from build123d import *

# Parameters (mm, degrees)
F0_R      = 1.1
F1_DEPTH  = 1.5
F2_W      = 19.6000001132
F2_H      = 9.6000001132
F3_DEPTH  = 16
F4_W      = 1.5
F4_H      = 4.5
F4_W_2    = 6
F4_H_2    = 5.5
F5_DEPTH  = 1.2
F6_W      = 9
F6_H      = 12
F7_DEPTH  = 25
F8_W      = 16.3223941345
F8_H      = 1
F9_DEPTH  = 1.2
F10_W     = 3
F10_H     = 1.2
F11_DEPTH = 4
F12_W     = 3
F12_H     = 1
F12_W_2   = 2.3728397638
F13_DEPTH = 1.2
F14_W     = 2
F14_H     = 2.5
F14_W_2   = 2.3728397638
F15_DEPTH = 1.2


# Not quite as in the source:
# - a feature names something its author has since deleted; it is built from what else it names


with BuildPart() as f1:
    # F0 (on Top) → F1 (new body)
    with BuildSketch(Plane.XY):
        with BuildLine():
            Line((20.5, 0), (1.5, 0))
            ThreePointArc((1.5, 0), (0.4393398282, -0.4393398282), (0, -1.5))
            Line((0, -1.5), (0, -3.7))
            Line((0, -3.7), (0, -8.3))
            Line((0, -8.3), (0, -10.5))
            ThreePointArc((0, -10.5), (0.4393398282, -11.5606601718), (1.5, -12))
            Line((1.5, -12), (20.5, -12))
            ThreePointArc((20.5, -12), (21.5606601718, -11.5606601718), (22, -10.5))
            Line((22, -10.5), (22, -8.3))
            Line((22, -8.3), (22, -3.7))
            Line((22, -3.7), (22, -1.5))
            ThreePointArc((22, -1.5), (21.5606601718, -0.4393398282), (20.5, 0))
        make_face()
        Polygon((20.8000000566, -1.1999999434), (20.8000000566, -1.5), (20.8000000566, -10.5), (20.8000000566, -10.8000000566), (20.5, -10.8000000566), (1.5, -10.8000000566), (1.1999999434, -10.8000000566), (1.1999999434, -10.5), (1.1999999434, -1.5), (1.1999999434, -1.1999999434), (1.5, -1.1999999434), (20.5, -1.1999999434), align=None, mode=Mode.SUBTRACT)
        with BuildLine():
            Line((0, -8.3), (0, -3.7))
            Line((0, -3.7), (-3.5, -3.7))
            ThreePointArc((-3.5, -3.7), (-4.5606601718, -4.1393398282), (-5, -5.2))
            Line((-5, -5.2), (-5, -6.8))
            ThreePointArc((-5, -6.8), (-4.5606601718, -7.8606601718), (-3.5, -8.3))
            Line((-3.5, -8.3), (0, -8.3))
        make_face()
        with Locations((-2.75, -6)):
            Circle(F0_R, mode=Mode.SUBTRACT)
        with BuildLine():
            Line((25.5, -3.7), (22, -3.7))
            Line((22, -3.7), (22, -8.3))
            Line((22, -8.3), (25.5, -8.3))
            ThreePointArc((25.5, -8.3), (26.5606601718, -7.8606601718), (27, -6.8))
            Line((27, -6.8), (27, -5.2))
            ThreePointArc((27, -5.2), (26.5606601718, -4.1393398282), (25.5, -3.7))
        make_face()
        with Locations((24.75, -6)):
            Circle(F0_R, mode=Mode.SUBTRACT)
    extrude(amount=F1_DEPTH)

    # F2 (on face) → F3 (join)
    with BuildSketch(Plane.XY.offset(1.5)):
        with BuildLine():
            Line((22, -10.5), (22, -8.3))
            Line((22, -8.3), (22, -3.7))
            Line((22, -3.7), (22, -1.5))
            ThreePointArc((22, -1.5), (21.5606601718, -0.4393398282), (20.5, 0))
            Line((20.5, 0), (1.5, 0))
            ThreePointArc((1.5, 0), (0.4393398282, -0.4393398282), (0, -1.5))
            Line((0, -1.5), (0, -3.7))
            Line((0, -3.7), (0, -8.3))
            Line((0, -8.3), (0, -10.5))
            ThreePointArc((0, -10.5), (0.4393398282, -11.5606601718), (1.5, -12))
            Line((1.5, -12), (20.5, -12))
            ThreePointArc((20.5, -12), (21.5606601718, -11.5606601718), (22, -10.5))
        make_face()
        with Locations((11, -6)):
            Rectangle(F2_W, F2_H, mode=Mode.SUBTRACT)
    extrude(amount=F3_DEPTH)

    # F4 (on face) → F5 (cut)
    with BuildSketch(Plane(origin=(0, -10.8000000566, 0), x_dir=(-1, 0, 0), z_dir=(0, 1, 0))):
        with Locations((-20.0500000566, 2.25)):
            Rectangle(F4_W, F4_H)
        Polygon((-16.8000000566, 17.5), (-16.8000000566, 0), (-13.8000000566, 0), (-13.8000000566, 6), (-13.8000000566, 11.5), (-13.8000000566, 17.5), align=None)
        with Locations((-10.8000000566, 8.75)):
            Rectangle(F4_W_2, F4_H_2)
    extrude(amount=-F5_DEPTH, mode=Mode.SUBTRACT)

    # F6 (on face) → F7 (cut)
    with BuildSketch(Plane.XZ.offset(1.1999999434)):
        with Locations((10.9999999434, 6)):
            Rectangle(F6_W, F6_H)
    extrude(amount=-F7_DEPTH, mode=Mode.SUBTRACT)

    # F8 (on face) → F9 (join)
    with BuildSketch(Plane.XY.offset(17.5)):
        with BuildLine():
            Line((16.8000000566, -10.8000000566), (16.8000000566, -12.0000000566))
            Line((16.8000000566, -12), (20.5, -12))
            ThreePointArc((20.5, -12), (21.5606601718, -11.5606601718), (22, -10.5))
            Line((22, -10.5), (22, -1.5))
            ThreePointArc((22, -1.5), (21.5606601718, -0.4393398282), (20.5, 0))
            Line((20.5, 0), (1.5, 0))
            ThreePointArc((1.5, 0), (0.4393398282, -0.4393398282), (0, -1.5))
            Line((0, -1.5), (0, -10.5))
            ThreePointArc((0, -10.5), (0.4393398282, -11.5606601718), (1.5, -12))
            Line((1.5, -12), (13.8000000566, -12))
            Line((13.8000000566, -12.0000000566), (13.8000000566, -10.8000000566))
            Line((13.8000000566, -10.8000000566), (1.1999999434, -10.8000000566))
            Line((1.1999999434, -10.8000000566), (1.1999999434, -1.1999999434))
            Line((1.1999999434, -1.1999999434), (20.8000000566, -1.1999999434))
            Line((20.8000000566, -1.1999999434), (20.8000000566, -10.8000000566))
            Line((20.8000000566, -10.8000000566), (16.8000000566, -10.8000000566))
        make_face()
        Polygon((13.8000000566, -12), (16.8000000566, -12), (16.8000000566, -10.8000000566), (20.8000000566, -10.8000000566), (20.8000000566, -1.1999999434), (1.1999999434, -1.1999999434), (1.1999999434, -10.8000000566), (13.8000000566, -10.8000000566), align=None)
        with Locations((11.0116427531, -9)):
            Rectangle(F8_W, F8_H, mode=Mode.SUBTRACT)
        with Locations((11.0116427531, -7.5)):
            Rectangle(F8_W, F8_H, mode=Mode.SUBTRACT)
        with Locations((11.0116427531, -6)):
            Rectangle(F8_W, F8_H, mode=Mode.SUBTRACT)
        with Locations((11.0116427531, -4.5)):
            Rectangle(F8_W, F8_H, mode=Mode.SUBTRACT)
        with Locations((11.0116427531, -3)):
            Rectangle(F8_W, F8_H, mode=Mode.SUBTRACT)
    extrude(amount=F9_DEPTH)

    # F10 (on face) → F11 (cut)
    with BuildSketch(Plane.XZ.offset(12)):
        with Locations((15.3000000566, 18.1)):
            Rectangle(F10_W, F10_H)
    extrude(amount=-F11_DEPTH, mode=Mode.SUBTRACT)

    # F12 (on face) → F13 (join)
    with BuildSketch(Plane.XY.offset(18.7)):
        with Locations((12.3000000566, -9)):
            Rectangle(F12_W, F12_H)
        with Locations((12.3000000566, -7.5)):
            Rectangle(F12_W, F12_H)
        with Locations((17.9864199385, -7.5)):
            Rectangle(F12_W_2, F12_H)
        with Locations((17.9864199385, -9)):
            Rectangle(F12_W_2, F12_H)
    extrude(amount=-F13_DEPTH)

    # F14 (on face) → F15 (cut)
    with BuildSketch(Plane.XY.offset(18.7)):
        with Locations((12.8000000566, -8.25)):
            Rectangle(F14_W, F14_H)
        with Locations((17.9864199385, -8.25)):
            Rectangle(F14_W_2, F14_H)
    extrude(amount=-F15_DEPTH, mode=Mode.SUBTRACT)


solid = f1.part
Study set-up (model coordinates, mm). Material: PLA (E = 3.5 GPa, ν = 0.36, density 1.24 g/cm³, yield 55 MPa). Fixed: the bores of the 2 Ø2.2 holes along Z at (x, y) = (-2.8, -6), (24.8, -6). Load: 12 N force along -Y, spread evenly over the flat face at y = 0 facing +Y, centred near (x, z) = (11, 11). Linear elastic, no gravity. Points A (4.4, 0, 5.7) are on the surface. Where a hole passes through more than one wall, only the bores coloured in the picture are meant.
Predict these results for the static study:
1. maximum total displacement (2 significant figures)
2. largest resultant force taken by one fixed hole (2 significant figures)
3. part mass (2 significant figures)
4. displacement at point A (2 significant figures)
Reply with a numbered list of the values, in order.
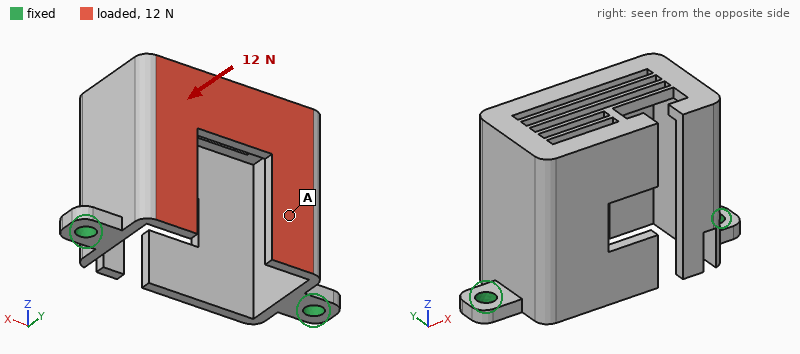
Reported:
1. 0.40 mm
2. 6.1 N
3. 1.6 g
4. 0.18 mm
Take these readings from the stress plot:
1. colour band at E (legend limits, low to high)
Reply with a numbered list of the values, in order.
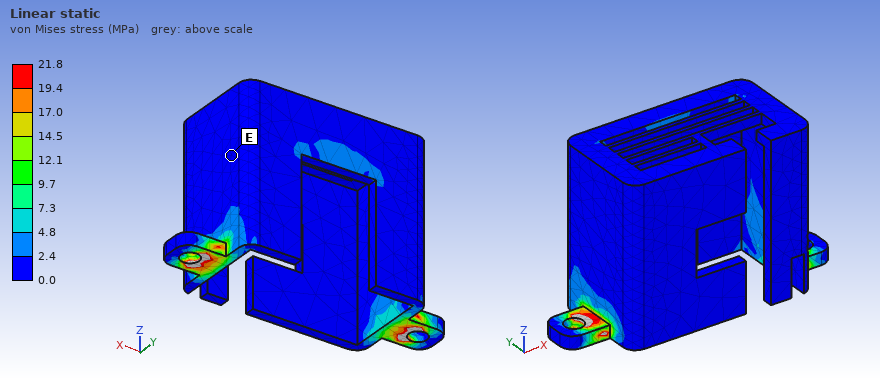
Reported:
1. 0.0 to 2.4 MPa
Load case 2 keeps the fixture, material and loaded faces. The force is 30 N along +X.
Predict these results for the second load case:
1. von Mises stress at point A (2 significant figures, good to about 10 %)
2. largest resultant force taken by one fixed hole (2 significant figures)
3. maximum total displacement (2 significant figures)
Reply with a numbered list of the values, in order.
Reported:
1. 3.2 MPa
2. 20 N
3. 0.23 mm
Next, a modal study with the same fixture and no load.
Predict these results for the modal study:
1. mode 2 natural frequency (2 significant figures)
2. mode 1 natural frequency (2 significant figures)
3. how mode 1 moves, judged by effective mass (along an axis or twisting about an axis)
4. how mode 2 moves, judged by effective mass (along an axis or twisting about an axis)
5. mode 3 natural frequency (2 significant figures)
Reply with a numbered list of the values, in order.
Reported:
1. 940 Hz
2. 780 Hz
3. along Y
4. along X
5. 1600 Hz
